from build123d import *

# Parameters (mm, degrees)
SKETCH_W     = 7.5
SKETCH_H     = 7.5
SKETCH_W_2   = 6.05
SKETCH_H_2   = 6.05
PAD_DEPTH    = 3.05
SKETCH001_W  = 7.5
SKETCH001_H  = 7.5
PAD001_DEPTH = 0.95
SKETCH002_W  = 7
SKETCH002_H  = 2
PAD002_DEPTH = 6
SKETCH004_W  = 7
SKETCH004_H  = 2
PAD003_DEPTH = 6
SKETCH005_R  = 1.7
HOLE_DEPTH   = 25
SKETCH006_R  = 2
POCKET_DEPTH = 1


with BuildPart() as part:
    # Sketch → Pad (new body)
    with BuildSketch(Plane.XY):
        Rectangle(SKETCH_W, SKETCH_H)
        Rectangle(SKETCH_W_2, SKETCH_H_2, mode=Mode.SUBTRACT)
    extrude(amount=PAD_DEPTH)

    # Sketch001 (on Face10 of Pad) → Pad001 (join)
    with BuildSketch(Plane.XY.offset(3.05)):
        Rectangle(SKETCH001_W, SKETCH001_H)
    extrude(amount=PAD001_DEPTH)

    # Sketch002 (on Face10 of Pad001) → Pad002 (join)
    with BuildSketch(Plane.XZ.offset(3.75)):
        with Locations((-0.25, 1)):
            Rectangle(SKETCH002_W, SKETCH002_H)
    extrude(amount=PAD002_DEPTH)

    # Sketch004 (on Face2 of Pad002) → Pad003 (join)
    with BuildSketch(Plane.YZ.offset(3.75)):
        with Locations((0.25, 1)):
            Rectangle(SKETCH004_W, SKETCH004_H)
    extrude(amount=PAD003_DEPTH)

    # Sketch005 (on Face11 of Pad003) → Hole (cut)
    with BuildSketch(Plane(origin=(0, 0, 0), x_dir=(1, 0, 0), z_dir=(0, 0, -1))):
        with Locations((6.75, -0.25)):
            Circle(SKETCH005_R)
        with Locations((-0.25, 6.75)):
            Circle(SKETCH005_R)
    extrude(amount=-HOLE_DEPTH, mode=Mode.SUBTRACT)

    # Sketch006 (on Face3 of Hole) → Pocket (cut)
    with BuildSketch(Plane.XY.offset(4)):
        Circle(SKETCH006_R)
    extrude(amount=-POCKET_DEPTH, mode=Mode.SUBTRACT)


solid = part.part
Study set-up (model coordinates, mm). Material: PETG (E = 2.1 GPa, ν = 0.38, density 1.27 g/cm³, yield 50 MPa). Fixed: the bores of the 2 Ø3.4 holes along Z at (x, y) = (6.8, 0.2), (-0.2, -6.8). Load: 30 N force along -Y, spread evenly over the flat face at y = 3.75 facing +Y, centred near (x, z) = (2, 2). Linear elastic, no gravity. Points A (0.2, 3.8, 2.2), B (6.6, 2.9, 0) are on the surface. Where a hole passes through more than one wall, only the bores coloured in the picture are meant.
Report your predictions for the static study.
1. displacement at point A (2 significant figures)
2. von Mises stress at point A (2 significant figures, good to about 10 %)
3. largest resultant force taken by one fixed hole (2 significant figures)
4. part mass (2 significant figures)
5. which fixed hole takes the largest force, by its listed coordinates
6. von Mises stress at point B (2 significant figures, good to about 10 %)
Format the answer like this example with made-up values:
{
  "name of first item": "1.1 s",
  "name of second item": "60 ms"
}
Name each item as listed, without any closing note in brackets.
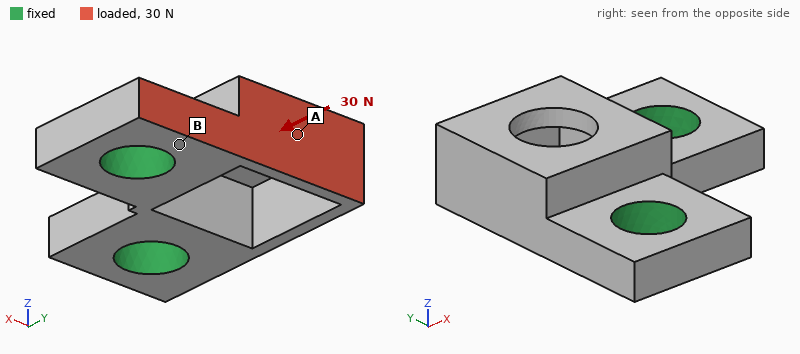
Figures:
{
  "displacement at point A": "44 µm",
  "von Mises stress at point A": "6.7 MPa",
  "largest resultant force taken by one fixed hole": "18 N",
  "part mass": "0.30 g",
  "which fixed hole takes the largest force, by its listed coordinates": "(6.8, 0.2)",
  "von Mises stress at point B": "2.3 MPa"
}
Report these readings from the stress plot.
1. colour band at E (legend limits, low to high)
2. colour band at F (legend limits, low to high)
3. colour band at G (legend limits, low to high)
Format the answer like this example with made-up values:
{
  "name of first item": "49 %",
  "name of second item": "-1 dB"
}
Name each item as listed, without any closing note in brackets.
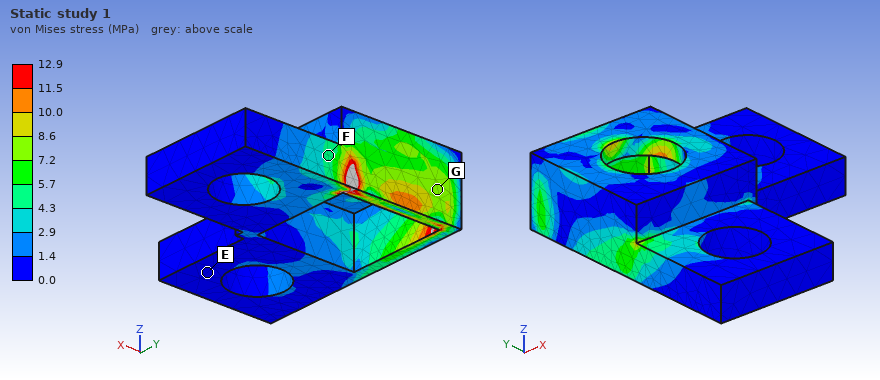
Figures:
{
  "colour band at E": "0.0 to 1.4 MPa",
  "colour band at F": "4.3 to 5.7 MPa",
  "colour band at G": "7.2 to 8.6 MPa"
}
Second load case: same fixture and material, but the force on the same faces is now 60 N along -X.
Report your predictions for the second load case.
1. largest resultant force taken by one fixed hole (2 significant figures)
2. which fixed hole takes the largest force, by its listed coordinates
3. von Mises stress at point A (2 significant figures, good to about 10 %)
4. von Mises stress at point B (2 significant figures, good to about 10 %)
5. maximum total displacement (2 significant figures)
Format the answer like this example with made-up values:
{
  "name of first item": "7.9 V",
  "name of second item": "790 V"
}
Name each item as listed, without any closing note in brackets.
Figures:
{
  "largest resultant force taken by one fixed hole": "59 N",
  "which fixed hole takes the largest force, by its listed coordinates": "(6.8, 0.2)",
  "von Mises stress at point A": "5.8 MPa",
  "von Mises stress at point B": "6.3 MPa",
  "maximum total displacement": "65 µm"
}
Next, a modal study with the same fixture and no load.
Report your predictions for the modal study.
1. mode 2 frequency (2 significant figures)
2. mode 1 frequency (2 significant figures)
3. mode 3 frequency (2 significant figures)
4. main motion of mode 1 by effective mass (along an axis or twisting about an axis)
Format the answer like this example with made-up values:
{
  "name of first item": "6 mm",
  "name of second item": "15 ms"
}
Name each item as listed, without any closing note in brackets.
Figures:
{
  "mode 2 frequency": "16 kHz",
  "mode 1 frequency": "7200 Hz",
  "mode 3 frequency": "22 kHz",
  "main motion of mode 1 by effective mass": "along Z"
}
